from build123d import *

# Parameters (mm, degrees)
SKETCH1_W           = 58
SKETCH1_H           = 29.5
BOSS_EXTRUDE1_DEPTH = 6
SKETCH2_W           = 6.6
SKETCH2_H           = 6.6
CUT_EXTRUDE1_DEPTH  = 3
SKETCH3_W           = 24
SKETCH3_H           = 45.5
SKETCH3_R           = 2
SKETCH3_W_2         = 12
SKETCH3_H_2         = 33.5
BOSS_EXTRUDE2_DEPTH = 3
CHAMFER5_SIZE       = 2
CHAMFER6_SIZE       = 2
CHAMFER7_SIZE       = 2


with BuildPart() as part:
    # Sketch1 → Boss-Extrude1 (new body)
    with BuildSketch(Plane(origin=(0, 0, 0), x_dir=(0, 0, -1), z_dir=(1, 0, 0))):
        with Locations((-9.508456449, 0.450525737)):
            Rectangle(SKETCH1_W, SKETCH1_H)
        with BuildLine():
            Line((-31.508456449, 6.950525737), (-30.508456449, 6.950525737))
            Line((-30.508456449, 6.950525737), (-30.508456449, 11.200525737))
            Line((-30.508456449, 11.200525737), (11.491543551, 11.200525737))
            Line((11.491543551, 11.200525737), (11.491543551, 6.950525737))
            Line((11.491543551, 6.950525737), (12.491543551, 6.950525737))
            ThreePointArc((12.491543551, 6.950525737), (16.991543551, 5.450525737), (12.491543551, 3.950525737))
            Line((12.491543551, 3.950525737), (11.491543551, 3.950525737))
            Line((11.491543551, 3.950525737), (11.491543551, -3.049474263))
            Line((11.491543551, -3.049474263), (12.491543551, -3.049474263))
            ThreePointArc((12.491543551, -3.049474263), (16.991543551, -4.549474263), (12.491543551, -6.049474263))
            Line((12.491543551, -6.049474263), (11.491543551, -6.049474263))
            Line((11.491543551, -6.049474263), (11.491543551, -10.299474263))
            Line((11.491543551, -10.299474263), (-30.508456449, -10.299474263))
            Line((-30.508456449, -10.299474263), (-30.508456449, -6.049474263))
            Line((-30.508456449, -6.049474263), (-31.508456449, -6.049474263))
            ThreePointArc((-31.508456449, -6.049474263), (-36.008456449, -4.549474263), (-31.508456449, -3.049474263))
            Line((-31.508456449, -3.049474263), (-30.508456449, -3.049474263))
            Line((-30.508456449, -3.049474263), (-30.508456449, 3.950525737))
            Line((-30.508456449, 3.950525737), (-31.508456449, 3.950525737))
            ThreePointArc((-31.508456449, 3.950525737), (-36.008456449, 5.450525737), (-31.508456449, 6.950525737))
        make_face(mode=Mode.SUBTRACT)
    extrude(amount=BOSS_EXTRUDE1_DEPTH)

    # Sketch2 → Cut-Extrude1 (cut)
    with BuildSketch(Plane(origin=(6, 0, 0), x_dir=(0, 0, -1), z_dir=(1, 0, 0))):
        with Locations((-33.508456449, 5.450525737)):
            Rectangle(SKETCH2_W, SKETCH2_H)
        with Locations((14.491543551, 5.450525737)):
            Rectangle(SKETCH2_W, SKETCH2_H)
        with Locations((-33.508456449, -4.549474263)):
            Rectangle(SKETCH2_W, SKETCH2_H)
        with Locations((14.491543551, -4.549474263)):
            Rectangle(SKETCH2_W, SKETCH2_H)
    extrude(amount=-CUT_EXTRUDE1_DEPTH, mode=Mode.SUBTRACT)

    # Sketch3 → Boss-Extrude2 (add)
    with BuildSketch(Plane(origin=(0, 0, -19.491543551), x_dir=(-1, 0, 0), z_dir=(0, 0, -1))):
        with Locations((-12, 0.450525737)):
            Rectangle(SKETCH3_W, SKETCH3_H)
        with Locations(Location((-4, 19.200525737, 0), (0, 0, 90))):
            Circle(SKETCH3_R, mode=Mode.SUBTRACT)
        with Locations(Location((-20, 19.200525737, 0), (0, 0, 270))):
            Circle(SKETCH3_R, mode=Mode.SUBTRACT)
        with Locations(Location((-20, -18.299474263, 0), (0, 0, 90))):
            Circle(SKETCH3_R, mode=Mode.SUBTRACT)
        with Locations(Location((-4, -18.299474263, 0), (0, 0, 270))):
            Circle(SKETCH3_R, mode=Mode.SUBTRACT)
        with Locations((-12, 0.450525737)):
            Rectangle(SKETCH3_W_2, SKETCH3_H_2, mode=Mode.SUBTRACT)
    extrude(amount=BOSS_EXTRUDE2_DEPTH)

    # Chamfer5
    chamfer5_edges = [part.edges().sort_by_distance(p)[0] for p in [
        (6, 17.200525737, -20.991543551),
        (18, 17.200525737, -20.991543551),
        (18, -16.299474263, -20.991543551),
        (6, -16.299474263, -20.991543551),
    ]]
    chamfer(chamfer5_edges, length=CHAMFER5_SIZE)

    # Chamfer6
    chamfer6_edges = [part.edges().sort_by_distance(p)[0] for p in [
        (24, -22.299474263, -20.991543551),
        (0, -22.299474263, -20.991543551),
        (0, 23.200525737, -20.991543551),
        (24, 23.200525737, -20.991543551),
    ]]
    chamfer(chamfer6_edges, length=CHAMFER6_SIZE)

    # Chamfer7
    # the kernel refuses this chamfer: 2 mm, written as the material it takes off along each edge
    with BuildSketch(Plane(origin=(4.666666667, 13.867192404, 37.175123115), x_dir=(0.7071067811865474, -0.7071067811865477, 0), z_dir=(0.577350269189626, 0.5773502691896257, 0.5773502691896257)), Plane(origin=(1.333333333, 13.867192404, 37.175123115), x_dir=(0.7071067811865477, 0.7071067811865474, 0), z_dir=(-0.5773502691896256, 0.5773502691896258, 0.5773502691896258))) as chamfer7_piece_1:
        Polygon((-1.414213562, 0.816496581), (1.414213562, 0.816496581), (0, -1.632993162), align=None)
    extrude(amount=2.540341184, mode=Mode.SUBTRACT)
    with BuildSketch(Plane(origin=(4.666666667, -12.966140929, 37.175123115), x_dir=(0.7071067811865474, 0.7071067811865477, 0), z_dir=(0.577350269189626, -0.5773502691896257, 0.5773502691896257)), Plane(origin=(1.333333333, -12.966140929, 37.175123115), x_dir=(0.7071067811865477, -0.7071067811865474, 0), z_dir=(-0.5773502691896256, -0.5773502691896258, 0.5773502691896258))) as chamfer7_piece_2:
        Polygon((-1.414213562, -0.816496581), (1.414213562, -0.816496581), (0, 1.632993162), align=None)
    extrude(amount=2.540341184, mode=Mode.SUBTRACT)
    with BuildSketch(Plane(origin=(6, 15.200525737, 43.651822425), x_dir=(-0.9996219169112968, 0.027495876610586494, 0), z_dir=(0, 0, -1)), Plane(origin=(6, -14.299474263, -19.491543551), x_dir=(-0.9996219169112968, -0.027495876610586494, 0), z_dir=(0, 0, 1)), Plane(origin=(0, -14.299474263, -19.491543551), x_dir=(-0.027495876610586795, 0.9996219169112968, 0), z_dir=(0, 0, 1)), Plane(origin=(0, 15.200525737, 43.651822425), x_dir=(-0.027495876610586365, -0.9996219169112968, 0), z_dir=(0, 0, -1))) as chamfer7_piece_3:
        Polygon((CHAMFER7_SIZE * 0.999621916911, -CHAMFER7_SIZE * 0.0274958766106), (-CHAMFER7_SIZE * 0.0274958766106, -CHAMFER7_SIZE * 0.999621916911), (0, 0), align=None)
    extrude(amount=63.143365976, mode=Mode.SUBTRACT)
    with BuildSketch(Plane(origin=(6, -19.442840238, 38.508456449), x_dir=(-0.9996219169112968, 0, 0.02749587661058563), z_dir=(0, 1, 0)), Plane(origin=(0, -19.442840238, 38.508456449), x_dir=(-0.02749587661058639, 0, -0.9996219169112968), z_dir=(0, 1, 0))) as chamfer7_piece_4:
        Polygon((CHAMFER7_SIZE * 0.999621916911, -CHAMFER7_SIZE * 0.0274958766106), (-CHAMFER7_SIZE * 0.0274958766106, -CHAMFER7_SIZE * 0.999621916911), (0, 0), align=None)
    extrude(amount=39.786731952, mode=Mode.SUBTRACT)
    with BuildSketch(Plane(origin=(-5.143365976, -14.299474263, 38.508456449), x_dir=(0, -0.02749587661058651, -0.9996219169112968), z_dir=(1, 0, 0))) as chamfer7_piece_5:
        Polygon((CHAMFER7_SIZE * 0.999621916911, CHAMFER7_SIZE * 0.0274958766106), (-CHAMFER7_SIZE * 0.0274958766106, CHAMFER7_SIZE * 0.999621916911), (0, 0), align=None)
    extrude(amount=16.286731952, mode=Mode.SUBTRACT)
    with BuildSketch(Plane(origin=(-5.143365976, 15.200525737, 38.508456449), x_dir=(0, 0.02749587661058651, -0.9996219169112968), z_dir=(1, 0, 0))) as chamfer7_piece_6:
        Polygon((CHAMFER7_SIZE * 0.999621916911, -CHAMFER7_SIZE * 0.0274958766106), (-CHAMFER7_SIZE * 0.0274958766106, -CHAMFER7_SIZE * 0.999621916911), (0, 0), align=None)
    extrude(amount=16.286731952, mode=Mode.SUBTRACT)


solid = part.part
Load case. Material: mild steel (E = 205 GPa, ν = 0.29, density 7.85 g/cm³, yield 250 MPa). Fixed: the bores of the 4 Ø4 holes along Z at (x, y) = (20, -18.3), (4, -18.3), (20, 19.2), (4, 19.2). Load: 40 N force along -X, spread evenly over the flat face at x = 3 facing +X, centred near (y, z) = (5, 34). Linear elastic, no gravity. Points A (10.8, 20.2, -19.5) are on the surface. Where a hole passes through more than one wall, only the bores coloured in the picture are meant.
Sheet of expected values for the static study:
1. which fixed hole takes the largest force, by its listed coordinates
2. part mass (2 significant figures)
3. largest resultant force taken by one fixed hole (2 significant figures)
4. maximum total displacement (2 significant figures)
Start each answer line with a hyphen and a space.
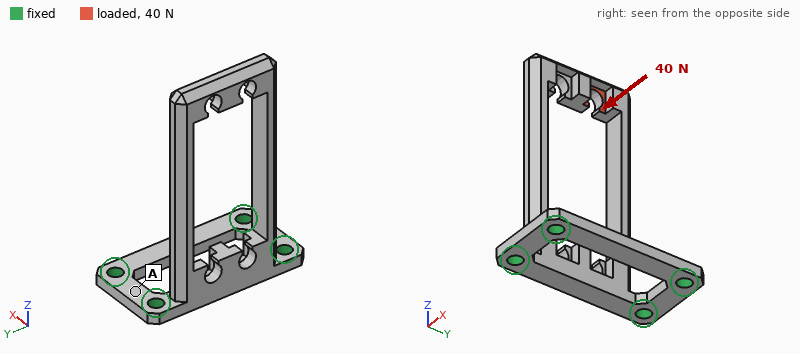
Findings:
- (4, 19.2)
- 43 g
- 25 N
- 0.18 mm
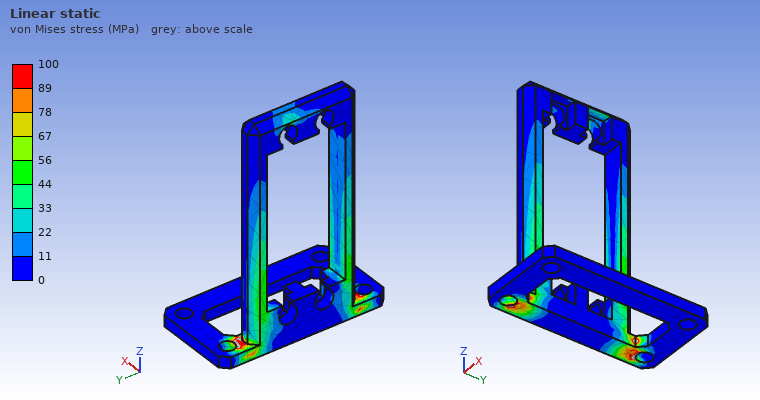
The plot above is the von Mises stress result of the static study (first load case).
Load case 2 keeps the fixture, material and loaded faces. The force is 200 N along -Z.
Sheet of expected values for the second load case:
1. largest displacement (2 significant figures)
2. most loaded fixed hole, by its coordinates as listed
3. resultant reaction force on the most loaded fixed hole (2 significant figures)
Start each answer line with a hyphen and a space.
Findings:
- 23 µm
- (4, 19.2)
- 130 N
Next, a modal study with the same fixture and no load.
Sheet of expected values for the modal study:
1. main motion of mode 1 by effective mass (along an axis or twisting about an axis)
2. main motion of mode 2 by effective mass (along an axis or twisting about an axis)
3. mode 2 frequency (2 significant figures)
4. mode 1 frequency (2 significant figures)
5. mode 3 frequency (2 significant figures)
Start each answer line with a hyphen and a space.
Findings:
- along X
- along Y
- 1300 Hz
- 790 Hz
- 2400 Hz
